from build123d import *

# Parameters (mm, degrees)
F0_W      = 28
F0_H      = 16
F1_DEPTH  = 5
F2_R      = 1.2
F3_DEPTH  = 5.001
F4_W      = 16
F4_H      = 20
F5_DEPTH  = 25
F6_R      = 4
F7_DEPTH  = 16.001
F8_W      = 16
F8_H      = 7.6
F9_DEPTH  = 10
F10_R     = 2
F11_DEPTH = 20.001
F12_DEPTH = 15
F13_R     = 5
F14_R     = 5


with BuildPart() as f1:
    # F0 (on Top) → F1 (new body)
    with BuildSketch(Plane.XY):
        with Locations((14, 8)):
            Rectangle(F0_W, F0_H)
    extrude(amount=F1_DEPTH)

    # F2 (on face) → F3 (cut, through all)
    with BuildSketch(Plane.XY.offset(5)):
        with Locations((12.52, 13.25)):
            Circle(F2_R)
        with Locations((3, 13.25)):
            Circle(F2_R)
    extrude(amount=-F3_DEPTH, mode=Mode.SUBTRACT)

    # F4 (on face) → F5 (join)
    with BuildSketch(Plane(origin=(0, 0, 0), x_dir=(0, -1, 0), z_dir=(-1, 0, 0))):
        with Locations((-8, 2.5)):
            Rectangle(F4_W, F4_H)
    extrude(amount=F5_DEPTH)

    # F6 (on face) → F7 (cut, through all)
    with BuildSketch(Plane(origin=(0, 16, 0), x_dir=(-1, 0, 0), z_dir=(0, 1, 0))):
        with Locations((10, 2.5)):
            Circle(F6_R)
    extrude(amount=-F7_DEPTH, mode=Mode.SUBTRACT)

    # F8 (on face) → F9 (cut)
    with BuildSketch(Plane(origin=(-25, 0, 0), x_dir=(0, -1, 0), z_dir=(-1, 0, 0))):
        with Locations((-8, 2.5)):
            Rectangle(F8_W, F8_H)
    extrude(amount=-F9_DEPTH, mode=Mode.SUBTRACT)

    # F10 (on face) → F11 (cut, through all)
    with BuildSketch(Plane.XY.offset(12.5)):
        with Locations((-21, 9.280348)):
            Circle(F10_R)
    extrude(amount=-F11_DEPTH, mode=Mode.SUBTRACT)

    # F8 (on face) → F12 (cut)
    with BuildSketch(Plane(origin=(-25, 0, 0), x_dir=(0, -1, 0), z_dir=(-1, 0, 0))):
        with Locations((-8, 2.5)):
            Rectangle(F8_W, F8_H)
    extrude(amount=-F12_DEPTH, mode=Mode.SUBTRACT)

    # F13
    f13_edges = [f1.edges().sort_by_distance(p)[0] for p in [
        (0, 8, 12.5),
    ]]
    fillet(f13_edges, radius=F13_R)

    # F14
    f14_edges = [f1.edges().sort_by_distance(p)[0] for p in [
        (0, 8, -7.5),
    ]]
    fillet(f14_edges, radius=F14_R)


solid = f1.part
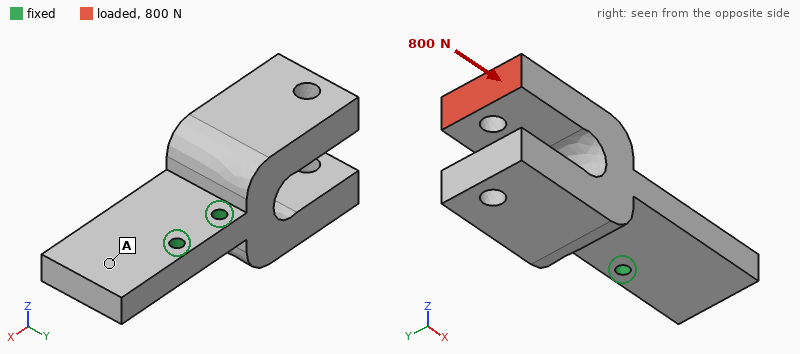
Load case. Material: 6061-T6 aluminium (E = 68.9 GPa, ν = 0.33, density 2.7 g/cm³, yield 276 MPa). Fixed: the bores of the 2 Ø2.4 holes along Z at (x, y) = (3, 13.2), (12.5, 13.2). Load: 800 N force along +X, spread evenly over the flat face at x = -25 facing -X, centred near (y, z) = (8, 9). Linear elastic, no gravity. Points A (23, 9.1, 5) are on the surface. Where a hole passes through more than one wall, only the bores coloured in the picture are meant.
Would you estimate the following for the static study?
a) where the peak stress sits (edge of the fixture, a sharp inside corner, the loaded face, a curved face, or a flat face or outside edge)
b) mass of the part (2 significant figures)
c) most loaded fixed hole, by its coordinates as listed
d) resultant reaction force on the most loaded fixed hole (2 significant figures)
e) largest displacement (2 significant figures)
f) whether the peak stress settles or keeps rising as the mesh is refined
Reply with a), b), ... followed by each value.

a) edge of the fixture
b) 21 g
c) (3, 13.2)
d) 680 N
e) 0.10 mm
f) keeps rising
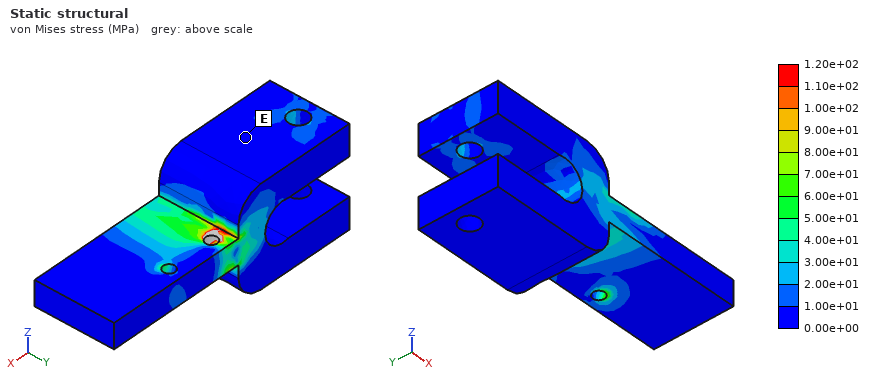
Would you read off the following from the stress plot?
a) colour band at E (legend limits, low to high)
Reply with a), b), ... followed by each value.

a) 0.00e+00 to 1.00e+01 MPa
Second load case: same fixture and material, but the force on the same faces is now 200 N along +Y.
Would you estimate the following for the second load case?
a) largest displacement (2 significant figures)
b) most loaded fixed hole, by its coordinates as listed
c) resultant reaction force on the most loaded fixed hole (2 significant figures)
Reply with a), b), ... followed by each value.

a) 39 µm
b) (3, 13.2)
c) 680 N
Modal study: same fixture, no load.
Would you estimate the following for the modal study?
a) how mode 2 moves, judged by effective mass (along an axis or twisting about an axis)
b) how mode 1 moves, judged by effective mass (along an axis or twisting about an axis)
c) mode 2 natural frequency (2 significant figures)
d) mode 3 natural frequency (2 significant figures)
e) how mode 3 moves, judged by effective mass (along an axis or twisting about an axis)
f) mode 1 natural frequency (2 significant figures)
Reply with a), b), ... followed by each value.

a) along Y
b) along Z
c) 6300 Hz
d) 7500 Hz
e) twisting about X
f) 3200 Hz
